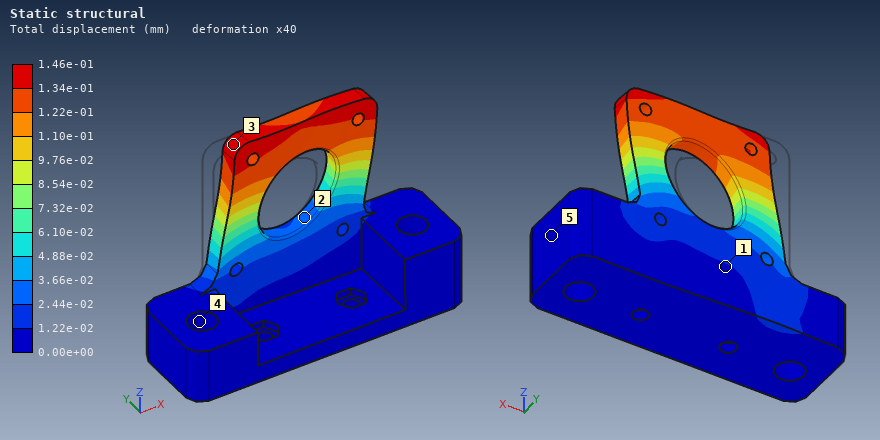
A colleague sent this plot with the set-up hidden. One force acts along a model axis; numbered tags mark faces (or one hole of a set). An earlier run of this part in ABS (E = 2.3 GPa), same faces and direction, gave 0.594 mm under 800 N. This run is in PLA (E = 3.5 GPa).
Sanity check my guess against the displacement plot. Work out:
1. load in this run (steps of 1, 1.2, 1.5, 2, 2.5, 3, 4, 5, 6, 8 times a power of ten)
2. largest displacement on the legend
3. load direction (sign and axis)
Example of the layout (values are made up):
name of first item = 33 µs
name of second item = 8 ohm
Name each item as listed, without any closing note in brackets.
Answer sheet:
load in this run = 300 N
largest displacement on the legend = 1.46e-01 mm
load direction = +X
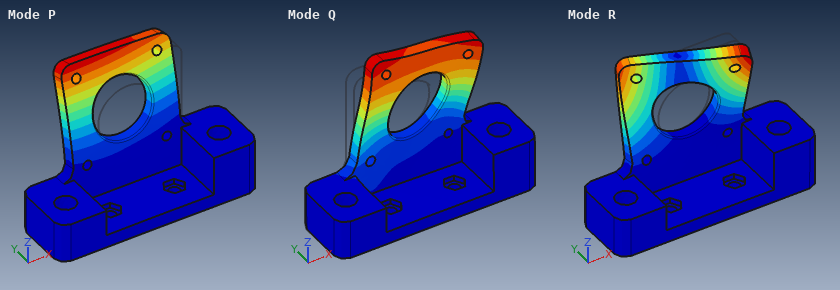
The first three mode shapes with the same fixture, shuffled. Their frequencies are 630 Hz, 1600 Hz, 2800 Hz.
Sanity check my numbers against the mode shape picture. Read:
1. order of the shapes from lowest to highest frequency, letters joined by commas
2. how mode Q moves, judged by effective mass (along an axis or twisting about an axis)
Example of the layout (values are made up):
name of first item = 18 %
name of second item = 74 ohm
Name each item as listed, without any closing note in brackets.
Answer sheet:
order of the shapes from lowest to highest frequency, letters joined by commas = P, R, Q
how mode Q moves, judged by effective mass = along X
